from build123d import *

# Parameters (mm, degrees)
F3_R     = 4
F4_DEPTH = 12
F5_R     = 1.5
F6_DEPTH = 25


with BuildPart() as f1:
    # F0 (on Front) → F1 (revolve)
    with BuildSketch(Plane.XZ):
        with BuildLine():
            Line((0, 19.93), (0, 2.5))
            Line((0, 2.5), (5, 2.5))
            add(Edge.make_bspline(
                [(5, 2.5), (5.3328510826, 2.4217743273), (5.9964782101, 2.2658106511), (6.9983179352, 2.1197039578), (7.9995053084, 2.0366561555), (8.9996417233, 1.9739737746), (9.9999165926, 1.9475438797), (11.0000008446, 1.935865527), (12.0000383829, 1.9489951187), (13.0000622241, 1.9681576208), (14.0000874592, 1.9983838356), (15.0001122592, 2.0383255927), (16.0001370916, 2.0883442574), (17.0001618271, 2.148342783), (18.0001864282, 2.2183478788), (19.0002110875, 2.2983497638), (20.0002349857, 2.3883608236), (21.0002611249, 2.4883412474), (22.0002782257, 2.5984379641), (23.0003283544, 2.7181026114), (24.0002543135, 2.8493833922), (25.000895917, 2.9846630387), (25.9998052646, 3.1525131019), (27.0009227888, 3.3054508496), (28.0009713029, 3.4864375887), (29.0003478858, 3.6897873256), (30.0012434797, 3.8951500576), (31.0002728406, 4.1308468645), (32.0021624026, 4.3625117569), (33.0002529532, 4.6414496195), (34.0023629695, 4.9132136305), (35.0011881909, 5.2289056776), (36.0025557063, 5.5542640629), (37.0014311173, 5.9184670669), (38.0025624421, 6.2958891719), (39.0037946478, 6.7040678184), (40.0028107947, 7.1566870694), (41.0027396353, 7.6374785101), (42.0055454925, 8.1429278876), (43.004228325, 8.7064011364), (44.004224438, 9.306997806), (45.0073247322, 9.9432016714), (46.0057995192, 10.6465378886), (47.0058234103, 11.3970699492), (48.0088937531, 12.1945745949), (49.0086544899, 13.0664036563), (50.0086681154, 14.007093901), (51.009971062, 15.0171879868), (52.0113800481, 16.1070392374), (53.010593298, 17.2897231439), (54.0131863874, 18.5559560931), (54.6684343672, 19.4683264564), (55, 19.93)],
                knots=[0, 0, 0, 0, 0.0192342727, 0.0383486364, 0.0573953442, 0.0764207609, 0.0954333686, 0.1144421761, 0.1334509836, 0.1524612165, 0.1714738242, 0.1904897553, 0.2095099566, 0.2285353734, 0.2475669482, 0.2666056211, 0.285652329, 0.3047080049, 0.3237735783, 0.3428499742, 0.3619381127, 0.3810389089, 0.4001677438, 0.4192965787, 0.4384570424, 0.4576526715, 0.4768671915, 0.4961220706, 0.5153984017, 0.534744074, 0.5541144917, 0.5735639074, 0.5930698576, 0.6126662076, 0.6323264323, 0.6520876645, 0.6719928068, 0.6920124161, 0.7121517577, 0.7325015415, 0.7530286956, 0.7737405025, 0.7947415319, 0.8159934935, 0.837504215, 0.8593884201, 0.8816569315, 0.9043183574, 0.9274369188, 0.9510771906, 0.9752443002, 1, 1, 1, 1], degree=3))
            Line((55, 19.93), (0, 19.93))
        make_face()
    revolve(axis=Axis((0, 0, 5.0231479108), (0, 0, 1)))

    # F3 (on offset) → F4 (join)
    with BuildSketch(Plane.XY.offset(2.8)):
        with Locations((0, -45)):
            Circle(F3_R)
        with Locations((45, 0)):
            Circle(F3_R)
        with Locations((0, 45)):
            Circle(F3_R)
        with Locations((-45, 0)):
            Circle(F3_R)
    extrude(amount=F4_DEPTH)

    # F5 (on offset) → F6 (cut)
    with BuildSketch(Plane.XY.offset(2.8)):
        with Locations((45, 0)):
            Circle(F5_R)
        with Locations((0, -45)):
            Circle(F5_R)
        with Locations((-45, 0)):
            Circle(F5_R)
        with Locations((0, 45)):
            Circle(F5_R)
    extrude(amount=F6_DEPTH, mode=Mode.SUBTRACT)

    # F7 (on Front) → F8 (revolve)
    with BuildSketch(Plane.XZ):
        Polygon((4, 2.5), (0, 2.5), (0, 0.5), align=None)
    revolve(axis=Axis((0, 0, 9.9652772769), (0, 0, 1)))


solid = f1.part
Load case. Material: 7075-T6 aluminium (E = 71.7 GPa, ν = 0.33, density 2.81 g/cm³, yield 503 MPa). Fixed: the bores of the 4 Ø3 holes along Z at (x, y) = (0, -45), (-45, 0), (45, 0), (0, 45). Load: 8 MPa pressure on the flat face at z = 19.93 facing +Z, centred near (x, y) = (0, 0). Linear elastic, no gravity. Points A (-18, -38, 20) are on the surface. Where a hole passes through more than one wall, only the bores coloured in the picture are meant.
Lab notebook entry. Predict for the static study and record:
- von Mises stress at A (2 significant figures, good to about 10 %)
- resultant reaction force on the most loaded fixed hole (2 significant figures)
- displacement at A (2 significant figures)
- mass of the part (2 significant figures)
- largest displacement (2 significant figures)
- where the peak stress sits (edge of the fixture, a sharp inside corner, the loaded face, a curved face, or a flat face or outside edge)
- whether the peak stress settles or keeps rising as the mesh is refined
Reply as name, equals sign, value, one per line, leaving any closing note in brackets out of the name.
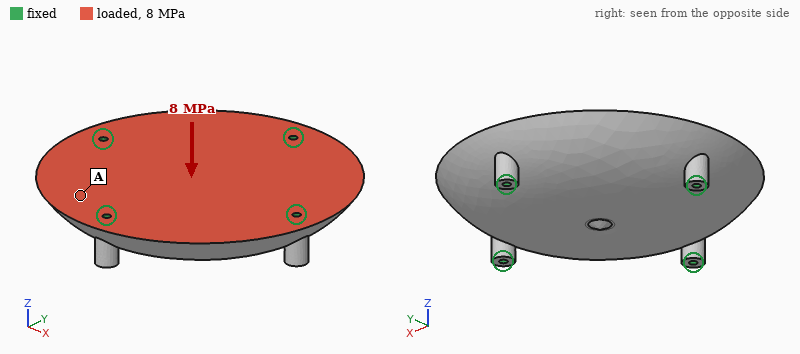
von Mises stress at A = 66 MPa
resultant reaction force on the most loaded fixed hole = 19 kN
displacement at A = 0.068 mm
mass of the part = 320 g
largest displacement = 0.12 mm
where the peak stress sits = edge of the fixture
whether the peak stress settles or keeps rising as the mesh is refined = keeps rising
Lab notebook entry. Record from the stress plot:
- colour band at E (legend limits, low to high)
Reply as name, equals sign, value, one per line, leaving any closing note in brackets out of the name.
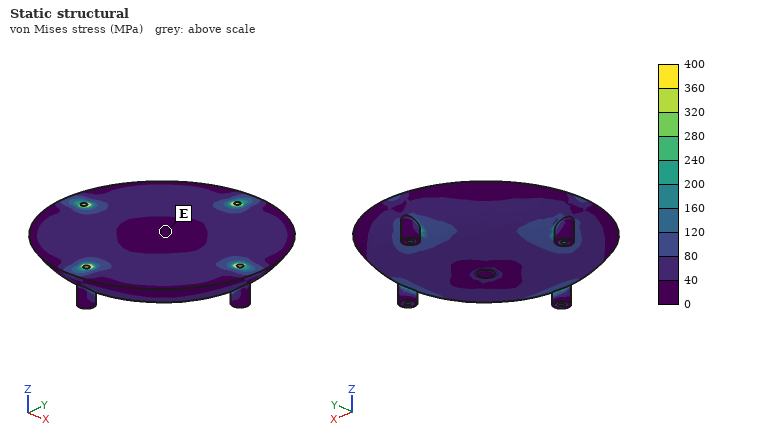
colour band at E = 0 to 40 MPa
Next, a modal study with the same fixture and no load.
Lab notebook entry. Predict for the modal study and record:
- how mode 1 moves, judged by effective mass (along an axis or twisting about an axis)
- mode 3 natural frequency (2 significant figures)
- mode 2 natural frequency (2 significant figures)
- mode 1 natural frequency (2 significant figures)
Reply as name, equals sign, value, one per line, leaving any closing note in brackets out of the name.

how mode 1 moves, judged by effective mass = along Z
mode 3 natural frequency = 10 kHz
mode 2 natural frequency = 10 kHz
mode 1 natural frequency = 8400 Hz
